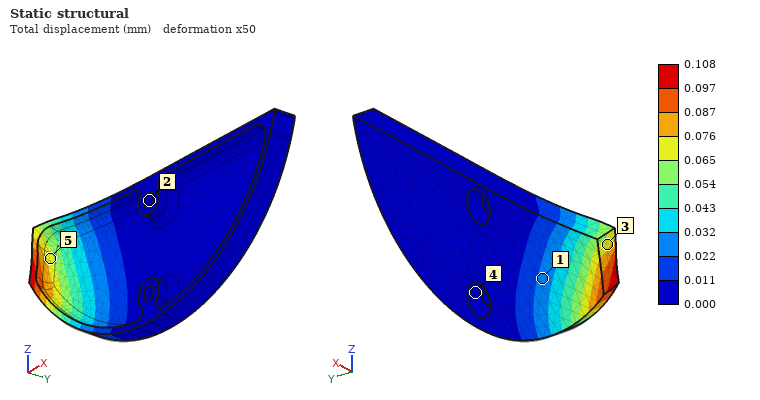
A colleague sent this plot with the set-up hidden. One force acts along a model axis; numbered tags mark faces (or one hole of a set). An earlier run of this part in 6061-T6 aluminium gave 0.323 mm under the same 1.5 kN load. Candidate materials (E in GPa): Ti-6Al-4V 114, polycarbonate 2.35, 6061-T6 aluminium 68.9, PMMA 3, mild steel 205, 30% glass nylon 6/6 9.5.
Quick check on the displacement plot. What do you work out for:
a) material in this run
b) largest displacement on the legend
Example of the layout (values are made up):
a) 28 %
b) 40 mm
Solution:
a) mild steel
b) 0.108 mm
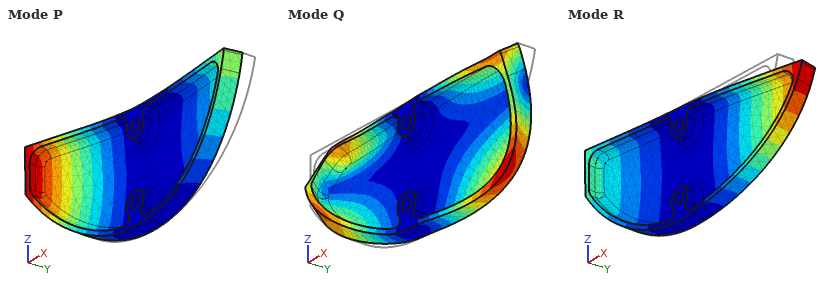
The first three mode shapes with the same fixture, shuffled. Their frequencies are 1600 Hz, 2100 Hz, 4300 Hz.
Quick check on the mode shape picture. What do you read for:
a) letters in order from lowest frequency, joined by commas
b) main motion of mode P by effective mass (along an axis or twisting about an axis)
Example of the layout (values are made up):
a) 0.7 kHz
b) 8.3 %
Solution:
a) R, P, Q
b) along Y
